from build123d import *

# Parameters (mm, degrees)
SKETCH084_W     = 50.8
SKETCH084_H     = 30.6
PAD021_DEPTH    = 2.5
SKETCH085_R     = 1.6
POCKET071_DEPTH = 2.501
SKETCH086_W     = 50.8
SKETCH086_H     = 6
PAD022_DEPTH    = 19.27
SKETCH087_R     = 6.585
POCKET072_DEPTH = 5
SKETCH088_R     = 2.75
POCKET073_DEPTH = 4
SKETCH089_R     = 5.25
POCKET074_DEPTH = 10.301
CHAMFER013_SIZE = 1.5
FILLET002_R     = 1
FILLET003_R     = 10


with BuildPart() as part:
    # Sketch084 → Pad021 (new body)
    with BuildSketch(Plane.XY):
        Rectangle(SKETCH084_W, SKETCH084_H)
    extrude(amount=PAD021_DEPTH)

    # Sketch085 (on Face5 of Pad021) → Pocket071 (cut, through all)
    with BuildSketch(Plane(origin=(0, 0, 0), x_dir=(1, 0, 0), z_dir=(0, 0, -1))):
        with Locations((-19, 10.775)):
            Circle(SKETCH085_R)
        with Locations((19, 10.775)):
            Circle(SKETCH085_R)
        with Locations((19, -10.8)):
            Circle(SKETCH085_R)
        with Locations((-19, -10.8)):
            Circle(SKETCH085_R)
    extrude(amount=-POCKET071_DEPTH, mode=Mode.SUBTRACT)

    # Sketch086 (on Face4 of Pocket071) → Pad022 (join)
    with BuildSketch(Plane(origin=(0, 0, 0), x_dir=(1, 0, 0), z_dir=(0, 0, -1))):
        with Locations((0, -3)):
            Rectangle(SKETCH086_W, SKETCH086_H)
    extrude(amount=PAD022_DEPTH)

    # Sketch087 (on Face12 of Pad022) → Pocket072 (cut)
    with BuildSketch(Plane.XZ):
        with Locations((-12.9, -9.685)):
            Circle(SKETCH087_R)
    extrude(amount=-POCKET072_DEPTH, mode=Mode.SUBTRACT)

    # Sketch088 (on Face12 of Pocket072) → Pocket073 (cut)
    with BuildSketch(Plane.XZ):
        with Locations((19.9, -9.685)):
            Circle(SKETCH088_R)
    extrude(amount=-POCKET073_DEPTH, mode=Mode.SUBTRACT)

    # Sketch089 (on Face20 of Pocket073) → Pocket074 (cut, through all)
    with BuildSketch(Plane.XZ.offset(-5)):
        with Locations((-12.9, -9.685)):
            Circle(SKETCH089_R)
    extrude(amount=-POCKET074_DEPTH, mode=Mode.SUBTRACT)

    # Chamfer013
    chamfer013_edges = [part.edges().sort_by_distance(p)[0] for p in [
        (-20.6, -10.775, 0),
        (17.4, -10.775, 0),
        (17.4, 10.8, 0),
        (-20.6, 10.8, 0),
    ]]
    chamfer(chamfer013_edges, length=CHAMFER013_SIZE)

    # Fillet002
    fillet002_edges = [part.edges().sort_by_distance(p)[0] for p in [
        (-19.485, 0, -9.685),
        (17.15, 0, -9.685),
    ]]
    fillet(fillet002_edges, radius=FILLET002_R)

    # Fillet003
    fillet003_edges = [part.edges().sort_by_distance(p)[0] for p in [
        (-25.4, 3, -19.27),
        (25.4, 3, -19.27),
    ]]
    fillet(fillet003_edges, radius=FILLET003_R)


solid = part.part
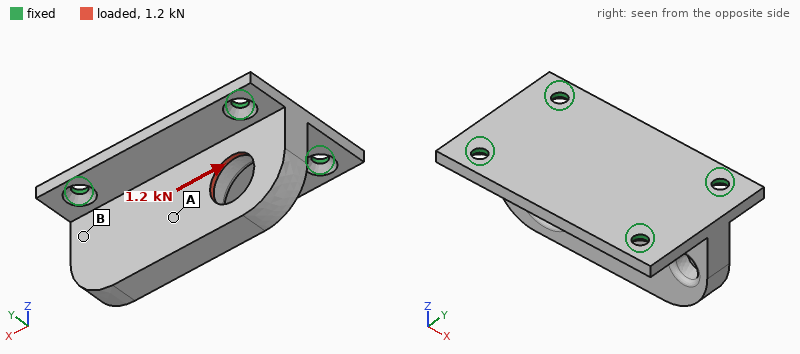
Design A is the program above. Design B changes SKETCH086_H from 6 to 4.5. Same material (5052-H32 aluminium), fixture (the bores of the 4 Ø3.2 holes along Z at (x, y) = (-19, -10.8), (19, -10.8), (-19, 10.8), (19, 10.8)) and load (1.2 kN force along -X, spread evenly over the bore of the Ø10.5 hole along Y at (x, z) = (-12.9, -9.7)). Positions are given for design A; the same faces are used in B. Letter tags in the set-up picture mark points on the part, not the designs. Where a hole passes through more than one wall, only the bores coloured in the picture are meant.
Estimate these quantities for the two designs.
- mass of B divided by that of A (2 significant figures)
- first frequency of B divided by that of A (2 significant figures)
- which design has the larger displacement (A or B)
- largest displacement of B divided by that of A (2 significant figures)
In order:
0.86
0.98
B
1.4
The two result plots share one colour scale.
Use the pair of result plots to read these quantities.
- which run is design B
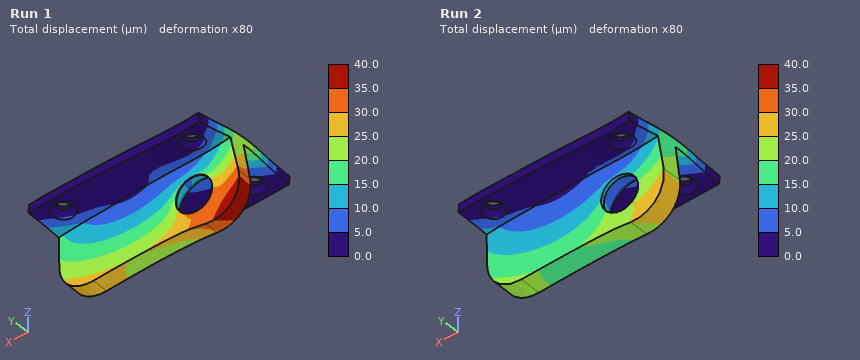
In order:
Run 1
